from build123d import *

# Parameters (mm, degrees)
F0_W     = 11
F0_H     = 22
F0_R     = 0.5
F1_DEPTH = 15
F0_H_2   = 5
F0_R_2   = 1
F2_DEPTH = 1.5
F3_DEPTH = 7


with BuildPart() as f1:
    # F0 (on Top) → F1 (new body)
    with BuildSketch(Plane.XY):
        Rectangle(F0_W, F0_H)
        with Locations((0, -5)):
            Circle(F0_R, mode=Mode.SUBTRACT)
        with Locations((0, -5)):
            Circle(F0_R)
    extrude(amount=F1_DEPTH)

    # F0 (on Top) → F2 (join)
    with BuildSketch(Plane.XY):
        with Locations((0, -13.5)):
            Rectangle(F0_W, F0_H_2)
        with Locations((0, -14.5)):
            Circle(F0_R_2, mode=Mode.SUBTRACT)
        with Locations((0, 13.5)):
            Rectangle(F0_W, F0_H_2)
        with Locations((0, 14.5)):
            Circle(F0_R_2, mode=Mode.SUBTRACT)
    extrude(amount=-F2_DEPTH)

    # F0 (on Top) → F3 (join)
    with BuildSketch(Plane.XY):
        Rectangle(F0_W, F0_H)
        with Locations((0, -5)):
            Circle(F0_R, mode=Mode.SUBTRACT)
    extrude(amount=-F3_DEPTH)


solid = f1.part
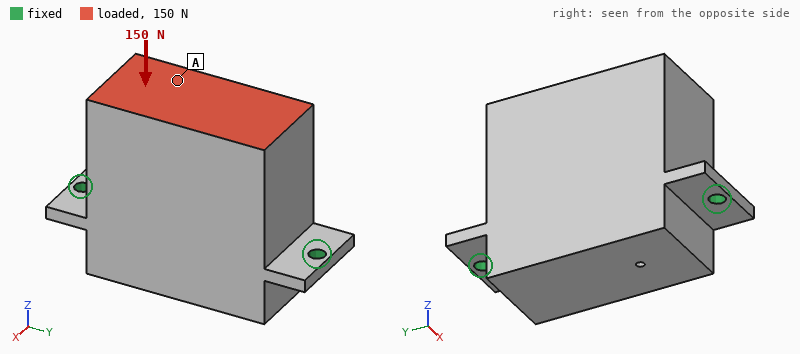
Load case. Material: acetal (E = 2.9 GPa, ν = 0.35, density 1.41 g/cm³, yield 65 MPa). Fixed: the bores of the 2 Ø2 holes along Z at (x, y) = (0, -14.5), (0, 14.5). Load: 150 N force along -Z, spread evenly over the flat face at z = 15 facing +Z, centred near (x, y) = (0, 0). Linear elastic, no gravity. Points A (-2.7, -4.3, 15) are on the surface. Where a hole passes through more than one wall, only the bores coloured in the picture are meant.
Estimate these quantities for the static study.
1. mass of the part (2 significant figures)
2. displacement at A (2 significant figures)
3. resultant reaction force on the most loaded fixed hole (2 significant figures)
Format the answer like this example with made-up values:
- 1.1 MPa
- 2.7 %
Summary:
- 7.7 g
- 77 µm
- 75 N
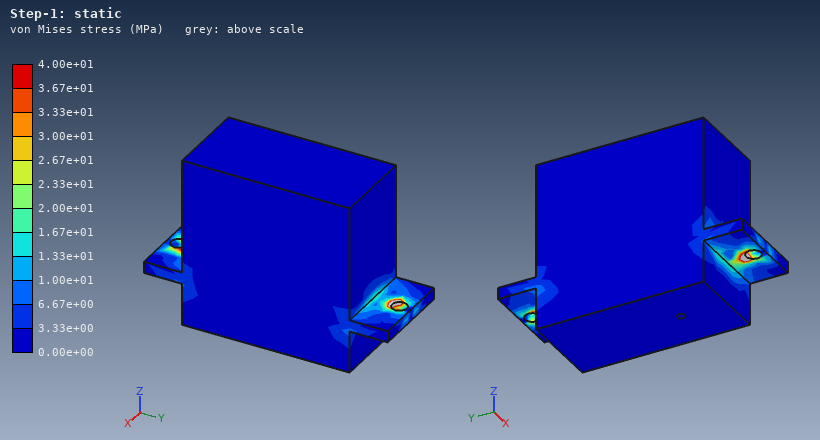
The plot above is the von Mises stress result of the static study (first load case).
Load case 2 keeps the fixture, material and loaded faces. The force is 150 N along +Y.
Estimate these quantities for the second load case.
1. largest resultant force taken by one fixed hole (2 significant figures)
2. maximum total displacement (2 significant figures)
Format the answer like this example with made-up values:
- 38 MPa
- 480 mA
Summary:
- 120 N
- 0.16 mm
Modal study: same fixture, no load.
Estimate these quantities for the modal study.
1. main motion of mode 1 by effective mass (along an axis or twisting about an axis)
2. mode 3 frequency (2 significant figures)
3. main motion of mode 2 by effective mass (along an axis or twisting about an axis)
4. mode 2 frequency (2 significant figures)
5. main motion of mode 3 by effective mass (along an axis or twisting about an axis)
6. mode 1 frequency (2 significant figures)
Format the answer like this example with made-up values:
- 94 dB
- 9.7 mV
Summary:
- along X
- 3100 Hz
- along Z
- 2600 Hz
- along Y
- 660 Hz
